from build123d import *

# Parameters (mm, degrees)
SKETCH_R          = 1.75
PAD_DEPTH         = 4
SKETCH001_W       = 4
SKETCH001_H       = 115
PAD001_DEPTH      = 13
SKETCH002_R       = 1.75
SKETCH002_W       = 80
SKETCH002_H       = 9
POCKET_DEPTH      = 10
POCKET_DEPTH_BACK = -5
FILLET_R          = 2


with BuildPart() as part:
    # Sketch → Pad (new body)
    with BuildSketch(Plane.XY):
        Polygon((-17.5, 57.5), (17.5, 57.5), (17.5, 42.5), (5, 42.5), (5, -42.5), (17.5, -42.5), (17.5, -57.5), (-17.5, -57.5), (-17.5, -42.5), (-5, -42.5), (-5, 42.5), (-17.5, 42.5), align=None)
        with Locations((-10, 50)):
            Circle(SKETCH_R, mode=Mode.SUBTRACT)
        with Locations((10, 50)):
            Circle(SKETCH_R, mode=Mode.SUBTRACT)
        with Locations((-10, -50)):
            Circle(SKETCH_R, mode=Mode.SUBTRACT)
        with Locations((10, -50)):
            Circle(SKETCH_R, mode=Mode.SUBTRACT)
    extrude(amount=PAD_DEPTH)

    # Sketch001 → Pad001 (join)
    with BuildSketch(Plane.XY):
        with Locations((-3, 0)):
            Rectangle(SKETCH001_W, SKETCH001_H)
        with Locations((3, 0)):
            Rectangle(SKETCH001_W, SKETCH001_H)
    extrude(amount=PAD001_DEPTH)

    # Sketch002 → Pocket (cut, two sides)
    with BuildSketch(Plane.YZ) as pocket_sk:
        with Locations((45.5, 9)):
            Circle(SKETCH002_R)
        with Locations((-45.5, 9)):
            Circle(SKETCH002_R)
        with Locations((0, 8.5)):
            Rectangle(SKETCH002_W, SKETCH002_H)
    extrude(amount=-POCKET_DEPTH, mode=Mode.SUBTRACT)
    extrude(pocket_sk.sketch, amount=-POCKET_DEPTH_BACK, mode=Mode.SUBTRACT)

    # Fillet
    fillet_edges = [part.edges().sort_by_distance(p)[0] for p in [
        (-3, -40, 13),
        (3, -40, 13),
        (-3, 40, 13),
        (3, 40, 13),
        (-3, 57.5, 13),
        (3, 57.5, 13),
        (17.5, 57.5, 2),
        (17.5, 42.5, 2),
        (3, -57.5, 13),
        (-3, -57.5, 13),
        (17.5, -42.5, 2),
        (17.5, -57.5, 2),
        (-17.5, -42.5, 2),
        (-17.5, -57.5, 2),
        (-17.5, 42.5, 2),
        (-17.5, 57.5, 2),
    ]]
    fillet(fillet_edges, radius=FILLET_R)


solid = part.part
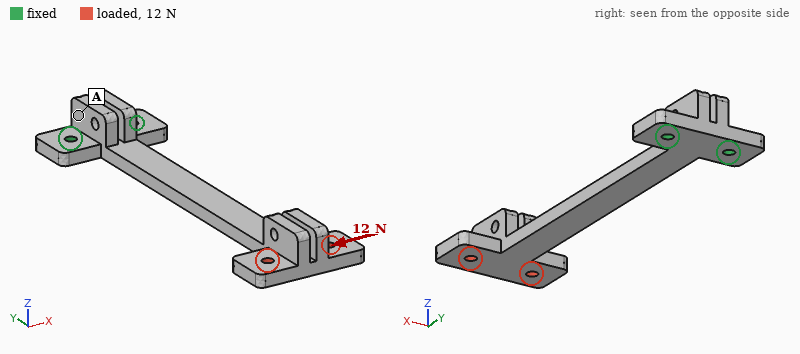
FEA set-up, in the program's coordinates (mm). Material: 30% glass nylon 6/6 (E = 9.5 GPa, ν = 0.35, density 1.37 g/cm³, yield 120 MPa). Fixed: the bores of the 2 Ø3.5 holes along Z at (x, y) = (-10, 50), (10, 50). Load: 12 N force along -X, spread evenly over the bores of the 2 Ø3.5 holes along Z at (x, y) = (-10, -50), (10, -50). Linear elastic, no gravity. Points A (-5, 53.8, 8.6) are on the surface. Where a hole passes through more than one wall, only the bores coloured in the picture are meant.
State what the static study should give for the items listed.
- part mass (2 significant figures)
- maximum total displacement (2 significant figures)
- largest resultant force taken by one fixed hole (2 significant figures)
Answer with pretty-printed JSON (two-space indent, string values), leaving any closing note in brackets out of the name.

{
  "part mass": "13 g",
  "maximum total displacement": "1.2 mm",
  "largest resultant force taken by one fixed hole": "63 N"
}
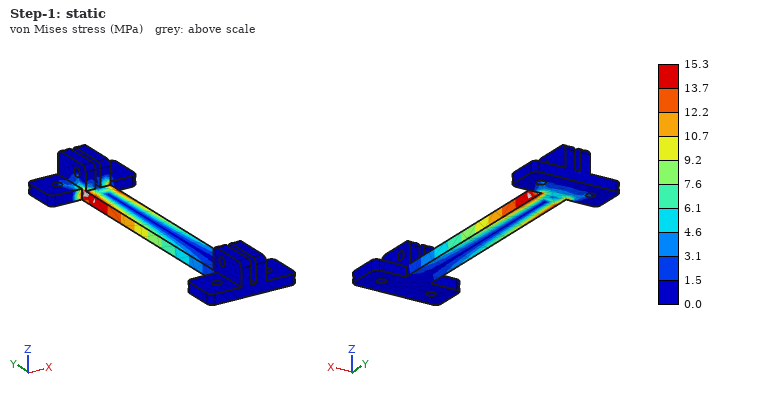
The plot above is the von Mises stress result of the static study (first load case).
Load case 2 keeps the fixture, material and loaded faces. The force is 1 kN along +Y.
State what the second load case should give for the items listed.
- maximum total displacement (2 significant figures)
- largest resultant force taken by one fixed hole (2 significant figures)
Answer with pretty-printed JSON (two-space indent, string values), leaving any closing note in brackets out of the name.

{
  "maximum total displacement": "0.38 mm",
  "largest resultant force taken by one fixed hole": "520 N"
}
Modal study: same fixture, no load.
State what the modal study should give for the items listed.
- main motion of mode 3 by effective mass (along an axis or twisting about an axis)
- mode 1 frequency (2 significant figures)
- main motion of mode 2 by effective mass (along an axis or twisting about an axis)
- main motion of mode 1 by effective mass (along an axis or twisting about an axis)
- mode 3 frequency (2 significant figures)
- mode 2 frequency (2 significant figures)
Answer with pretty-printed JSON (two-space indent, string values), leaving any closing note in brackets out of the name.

{
  "main motion of mode 3 by effective mass": "twisting about Y",
  "mode 1 frequency": "94 Hz",
  "main motion of mode 2 by effective mass": "along X",
  "main motion of mode 1 by effective mass": "along Z",
  "mode 3 frequency": "690 Hz",
  "mode 2 frequency": "230 Hz"
}
